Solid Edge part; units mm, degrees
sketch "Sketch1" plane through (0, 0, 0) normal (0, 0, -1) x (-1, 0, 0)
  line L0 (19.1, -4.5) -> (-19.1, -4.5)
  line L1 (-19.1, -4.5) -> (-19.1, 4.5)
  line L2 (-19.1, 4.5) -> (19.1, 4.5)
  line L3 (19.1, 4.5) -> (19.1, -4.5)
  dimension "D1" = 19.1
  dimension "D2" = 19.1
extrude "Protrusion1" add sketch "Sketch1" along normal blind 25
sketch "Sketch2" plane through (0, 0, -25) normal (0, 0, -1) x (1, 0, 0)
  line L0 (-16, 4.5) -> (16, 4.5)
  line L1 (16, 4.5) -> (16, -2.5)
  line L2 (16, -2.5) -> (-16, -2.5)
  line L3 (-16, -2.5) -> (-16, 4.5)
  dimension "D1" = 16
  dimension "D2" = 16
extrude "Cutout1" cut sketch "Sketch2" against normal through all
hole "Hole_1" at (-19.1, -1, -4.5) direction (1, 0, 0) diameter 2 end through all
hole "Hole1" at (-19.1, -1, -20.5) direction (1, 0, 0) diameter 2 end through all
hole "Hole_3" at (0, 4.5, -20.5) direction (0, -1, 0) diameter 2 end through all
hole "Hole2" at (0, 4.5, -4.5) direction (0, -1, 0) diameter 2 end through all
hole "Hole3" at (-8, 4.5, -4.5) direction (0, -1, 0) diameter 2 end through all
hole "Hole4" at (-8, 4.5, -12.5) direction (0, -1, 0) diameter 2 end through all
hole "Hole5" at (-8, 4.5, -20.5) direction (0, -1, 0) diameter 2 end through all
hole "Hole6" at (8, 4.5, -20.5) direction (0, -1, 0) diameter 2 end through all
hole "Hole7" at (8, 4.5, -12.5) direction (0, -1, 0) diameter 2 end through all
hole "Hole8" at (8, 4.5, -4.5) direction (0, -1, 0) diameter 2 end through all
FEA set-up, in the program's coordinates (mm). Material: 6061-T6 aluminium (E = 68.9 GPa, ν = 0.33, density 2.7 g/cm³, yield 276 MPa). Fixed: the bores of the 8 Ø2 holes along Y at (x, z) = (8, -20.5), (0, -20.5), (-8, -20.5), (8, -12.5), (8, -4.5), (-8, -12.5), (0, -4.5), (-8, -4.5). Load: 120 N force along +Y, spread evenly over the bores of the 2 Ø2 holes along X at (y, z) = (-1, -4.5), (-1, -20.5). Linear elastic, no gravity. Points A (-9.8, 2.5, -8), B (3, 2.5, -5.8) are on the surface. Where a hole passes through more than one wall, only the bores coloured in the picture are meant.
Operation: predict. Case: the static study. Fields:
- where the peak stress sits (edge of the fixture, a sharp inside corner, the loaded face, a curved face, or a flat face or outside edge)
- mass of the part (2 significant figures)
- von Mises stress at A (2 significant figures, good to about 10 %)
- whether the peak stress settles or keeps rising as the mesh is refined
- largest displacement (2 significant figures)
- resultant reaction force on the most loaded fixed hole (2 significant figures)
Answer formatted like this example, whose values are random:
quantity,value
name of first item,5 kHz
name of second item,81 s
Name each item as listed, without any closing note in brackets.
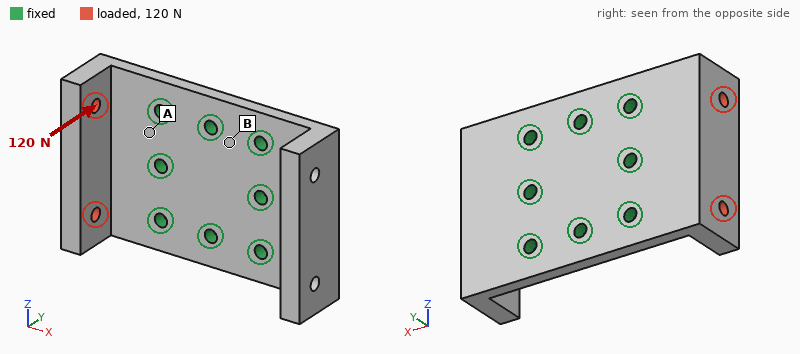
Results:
quantity,value
where the peak stress sits,edge of the fixture
mass of the part,7.8 g
von Mises stress at A,39 MPa
whether the peak stress settles or keeps rising as the mesh is refined,keeps rising
largest displacement,49 µm
resultant reaction force on the most loaded fixed hole,51 N
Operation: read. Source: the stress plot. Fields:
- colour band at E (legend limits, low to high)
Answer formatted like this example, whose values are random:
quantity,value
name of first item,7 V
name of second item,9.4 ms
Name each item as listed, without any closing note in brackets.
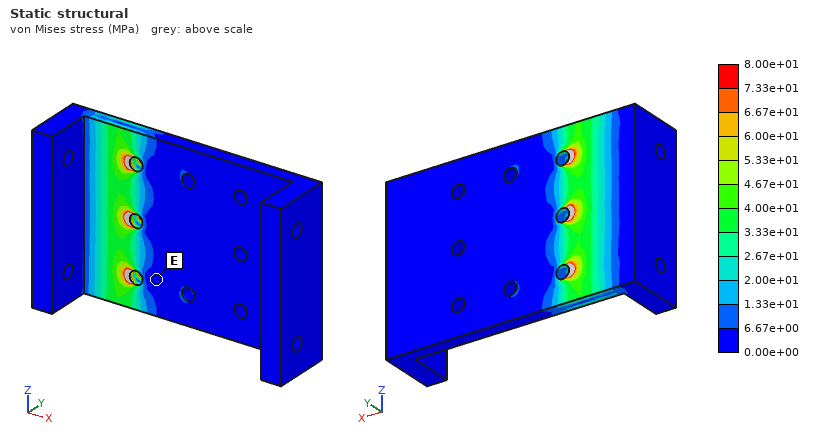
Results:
quantity,value
colour band at E,0.00e+00 to 6.67e+00 MPa
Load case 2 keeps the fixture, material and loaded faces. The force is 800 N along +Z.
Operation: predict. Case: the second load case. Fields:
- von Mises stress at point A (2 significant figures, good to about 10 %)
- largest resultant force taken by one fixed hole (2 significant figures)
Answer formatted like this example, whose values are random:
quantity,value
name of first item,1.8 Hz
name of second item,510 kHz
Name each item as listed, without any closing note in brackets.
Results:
quantity,value
von Mises stress at point A,70 MPa
largest resultant force taken by one fixed hole,480 N
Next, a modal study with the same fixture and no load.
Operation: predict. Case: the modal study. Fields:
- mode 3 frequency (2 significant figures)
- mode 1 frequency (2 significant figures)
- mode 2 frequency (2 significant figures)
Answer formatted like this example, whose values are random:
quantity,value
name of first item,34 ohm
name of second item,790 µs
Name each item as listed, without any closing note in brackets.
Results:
quantity,value
mode 3 frequency,11 kHz
mode 1 frequency,6100 Hz
mode 2 frequency,6100 Hz
